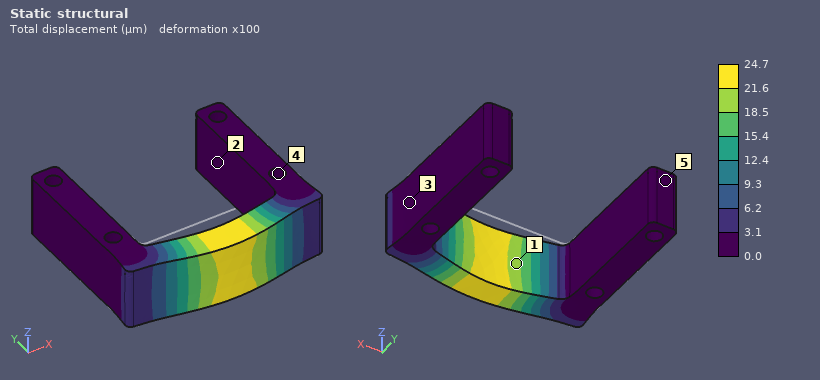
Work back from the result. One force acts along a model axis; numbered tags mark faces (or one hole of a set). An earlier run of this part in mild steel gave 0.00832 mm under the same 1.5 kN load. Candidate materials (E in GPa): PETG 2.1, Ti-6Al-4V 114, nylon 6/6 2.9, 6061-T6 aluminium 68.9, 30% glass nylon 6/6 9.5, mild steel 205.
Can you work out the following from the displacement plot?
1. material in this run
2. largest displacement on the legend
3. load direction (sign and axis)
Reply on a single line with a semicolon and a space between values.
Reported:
6061-T6 aluminium; 24.7 µm; -Y
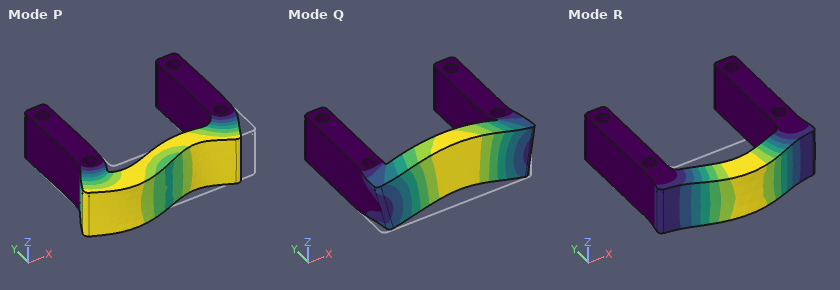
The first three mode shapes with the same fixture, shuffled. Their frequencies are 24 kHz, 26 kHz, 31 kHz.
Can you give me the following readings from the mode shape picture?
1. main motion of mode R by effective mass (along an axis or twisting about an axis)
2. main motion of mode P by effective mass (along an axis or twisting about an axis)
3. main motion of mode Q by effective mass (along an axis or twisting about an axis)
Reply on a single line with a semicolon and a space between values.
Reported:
along Y; along X; along Z
